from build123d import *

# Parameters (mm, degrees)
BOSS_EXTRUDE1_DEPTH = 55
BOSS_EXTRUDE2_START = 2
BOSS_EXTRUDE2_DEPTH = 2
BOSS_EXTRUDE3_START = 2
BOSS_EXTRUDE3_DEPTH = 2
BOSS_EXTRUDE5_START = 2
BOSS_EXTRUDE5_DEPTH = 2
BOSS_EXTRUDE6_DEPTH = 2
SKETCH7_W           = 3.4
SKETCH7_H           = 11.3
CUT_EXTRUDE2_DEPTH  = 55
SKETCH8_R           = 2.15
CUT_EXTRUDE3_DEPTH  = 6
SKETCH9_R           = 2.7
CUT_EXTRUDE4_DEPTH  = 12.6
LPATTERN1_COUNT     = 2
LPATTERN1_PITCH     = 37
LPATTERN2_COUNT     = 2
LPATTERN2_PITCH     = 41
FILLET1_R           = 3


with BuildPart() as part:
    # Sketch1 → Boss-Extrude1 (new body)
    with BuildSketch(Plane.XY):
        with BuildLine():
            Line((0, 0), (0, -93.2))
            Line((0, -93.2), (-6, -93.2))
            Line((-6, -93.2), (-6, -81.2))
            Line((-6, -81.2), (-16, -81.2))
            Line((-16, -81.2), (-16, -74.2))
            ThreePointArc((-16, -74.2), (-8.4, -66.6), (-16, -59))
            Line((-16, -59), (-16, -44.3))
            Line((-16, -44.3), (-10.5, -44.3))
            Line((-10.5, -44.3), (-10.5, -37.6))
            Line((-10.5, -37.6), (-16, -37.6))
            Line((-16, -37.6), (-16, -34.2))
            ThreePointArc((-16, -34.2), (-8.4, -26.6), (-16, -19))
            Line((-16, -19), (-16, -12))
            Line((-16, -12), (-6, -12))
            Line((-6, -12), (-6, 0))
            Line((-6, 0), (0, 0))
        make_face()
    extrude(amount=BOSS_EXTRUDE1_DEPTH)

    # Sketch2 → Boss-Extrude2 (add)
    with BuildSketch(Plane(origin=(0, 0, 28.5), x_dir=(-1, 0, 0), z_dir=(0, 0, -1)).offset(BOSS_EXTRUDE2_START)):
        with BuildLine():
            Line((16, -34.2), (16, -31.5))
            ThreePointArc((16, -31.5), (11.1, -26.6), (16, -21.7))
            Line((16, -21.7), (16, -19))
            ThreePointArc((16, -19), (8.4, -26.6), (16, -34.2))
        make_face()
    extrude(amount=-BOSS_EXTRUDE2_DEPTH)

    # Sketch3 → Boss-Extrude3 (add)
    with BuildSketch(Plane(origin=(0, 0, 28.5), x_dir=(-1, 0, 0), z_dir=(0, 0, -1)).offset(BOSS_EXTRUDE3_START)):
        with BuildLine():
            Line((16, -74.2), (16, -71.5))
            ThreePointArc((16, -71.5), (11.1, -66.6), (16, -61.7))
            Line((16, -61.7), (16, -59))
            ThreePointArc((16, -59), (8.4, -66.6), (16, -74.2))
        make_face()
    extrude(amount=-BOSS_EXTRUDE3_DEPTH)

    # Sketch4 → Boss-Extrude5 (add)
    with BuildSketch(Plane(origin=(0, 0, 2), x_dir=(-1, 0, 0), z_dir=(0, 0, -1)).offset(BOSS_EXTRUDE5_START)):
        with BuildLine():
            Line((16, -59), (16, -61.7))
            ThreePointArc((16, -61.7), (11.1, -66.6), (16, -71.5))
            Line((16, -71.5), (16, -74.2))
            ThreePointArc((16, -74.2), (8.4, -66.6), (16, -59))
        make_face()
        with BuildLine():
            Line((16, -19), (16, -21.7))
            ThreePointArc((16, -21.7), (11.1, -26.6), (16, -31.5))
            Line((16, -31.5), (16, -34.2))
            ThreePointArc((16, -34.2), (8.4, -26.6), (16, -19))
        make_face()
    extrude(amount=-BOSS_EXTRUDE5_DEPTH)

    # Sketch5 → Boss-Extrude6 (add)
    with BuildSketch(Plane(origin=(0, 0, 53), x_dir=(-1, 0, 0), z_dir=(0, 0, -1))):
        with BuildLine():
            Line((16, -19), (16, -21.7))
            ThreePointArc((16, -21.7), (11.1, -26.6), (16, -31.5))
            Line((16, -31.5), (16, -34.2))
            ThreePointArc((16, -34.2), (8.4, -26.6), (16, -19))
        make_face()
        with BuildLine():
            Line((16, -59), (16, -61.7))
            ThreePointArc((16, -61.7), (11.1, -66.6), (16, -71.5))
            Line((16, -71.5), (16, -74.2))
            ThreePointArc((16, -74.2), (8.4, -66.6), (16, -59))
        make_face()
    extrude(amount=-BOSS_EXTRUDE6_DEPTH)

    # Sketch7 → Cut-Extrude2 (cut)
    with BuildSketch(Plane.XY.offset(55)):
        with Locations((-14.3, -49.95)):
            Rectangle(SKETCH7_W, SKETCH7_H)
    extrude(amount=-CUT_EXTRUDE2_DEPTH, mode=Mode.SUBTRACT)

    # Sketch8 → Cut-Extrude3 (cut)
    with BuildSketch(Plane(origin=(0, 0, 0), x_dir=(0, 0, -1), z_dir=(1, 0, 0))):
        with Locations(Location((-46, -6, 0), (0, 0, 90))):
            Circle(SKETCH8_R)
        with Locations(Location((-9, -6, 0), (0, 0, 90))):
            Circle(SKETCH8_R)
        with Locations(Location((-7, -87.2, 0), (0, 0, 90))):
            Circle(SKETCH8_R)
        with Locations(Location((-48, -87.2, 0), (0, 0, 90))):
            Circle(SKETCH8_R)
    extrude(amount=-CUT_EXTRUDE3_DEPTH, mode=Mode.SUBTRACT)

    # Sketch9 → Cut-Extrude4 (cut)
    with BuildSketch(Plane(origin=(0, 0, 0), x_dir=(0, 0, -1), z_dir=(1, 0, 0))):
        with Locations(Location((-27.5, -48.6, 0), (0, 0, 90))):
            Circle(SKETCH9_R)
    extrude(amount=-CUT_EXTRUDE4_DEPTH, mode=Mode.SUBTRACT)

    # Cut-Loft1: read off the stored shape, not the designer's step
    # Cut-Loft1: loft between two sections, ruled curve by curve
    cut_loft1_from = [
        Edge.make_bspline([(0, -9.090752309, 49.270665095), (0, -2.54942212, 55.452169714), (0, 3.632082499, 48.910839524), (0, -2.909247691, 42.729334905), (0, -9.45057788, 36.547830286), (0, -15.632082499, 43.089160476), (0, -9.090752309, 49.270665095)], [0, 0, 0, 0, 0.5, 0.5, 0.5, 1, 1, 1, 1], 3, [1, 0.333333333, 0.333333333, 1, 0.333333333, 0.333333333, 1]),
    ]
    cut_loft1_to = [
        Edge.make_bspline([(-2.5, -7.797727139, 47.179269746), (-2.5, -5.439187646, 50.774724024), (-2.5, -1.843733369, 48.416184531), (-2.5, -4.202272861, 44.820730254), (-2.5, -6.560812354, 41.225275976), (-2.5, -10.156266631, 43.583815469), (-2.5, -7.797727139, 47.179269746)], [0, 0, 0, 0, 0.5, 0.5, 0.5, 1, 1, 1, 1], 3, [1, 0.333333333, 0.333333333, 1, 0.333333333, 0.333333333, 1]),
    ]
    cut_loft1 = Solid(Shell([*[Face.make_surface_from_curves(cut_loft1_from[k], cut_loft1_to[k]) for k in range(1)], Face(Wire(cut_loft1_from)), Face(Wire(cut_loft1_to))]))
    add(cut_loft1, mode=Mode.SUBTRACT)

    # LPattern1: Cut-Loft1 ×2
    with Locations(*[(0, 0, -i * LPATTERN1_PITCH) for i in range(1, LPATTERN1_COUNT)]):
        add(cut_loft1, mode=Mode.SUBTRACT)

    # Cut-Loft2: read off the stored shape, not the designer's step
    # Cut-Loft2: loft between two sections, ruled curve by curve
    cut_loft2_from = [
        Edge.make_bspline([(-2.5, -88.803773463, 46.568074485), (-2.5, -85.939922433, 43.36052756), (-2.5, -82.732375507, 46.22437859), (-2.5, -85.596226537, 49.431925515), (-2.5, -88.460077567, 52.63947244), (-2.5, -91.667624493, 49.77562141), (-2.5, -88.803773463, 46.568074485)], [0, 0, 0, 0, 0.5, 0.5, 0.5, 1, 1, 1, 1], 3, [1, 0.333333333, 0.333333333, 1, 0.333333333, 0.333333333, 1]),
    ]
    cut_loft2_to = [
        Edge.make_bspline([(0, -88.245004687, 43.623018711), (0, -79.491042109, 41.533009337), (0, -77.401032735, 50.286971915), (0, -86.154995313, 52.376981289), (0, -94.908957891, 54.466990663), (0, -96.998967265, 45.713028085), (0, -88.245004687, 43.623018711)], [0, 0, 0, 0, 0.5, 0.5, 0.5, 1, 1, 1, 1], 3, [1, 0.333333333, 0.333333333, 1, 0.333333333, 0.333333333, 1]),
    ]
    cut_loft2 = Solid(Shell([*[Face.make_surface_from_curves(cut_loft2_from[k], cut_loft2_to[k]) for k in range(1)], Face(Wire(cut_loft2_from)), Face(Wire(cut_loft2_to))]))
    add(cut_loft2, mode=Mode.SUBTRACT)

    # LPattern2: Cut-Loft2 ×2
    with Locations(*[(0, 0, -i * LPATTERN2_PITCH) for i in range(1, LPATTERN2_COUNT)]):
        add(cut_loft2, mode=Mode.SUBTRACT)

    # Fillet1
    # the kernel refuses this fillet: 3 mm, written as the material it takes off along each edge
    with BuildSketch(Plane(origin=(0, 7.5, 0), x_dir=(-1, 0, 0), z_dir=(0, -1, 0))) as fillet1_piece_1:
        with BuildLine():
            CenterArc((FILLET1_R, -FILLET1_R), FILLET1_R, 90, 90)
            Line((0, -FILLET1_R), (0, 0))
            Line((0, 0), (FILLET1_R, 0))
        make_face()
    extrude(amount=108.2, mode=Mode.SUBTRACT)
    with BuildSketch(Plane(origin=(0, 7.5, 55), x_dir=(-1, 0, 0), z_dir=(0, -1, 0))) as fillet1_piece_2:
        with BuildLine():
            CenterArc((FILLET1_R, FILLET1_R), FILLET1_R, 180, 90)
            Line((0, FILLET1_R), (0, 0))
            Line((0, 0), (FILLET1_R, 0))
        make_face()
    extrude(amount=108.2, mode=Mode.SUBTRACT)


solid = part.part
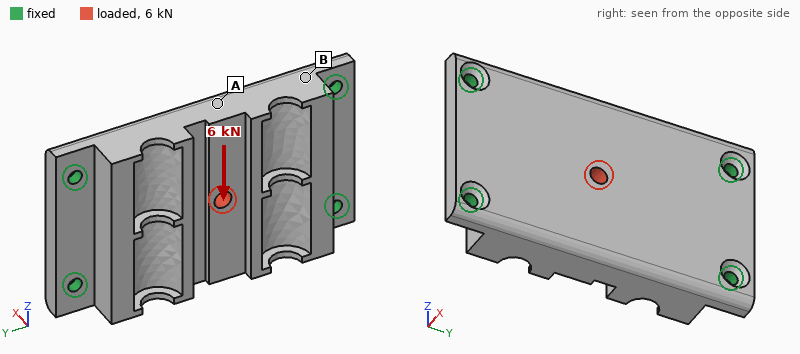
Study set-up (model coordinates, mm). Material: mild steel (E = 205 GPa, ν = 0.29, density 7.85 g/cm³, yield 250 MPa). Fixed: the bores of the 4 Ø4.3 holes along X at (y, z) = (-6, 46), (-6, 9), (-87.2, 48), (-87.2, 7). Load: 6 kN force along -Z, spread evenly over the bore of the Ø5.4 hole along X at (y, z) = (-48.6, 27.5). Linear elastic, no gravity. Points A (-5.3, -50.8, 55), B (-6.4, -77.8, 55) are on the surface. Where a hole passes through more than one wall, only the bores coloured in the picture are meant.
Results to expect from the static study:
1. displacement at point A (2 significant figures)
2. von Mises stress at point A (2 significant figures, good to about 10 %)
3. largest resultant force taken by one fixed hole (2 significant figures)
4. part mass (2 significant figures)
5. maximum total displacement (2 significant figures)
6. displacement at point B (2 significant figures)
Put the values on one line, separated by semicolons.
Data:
5.4 µm; 16 MPa; 2.0 kN; 420 g; 6.6 µm; 2.8 µm
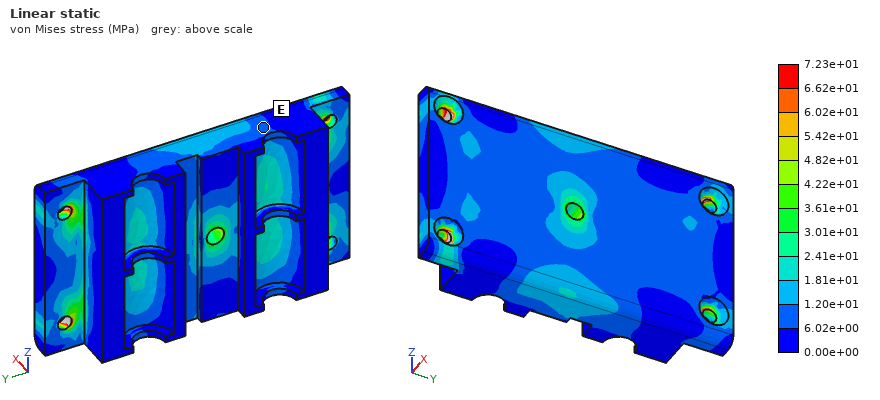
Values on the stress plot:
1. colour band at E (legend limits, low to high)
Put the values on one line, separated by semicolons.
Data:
6.02e+00 to 1.20e+01 MPa
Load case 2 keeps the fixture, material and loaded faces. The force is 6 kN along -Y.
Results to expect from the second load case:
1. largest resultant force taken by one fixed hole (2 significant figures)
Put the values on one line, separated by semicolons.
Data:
1.5 kN
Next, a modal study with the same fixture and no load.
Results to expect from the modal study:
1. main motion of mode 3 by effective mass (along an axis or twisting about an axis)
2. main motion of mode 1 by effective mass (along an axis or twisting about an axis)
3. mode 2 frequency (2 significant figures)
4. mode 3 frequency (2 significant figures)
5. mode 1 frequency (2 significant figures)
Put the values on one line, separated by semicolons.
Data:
twisting about Z; along X; 6800 Hz; 12 kHz; 4300 Hz
